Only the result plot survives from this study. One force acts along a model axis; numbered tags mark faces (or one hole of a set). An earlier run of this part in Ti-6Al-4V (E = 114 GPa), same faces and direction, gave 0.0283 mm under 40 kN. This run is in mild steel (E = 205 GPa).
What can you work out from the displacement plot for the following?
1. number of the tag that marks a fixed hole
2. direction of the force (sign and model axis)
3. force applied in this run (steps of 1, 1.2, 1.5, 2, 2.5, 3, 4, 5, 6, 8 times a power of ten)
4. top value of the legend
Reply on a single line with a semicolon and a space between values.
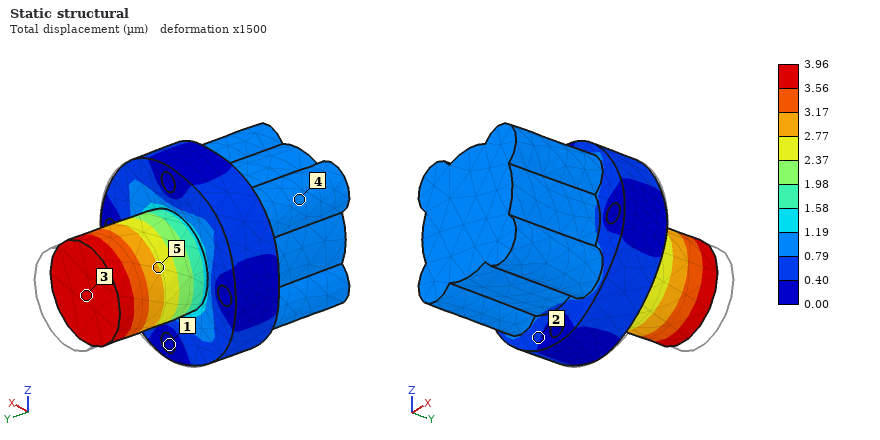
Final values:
1; -Y; 10 kN; 3.96 µm
